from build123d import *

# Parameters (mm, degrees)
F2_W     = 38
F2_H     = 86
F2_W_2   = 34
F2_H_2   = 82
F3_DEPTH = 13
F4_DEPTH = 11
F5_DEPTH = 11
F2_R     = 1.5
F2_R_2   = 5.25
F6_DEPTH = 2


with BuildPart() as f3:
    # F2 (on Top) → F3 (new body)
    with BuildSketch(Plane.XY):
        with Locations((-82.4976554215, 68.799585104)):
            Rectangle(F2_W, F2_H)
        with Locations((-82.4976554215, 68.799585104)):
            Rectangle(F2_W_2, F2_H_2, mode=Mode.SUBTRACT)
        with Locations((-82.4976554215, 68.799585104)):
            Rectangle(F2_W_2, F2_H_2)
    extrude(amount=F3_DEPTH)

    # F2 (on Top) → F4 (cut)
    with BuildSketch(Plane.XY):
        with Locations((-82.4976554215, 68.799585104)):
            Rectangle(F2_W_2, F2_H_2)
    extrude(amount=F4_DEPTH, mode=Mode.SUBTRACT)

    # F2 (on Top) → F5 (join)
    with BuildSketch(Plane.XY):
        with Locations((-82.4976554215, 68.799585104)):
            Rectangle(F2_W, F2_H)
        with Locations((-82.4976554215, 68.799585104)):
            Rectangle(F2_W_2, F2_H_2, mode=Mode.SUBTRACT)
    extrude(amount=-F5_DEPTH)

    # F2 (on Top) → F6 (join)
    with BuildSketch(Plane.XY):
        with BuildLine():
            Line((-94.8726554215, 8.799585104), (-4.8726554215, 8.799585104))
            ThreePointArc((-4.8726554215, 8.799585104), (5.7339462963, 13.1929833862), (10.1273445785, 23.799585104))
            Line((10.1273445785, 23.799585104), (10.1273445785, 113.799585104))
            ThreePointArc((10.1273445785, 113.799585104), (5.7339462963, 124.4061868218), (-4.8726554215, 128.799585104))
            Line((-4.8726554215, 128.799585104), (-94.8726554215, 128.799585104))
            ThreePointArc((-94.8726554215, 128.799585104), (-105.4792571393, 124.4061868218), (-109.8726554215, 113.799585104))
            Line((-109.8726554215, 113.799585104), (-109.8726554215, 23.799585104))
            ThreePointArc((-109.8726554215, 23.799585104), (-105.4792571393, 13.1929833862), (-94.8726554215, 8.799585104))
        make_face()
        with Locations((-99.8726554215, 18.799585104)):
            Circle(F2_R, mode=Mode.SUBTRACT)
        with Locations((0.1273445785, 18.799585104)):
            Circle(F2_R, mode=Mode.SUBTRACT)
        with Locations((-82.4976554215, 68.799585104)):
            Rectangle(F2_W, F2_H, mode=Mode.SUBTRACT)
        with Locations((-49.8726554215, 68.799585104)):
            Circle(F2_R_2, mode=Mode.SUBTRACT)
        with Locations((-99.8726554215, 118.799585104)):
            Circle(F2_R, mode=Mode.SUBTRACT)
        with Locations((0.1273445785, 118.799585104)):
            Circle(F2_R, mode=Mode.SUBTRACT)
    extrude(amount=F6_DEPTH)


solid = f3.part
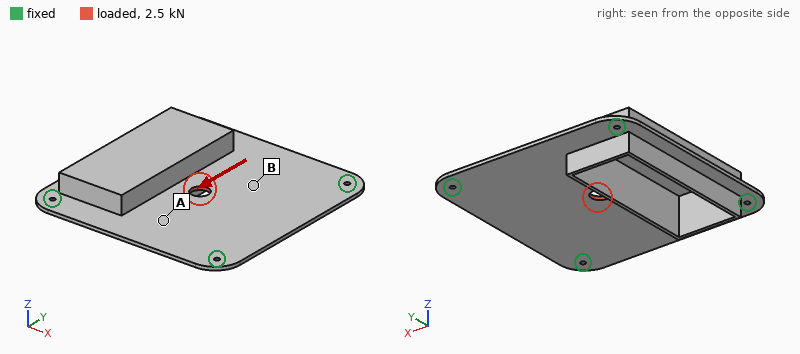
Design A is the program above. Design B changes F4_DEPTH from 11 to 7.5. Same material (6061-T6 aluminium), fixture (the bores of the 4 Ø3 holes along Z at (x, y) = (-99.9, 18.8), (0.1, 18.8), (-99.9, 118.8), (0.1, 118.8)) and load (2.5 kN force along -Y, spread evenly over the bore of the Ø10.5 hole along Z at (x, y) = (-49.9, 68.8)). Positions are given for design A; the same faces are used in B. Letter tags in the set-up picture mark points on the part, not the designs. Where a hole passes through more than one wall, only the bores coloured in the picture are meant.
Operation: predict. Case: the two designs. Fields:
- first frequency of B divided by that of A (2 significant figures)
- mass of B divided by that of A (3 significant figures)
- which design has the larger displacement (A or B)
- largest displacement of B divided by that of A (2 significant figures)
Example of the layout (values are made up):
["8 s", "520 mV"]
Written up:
["0.93", "1.25", "A", "0.90"]
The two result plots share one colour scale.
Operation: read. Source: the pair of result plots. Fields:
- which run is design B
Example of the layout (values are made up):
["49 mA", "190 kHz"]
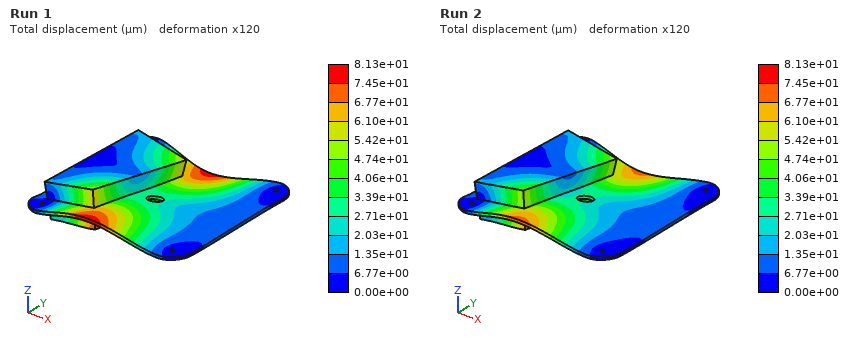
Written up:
["Run 2"]
